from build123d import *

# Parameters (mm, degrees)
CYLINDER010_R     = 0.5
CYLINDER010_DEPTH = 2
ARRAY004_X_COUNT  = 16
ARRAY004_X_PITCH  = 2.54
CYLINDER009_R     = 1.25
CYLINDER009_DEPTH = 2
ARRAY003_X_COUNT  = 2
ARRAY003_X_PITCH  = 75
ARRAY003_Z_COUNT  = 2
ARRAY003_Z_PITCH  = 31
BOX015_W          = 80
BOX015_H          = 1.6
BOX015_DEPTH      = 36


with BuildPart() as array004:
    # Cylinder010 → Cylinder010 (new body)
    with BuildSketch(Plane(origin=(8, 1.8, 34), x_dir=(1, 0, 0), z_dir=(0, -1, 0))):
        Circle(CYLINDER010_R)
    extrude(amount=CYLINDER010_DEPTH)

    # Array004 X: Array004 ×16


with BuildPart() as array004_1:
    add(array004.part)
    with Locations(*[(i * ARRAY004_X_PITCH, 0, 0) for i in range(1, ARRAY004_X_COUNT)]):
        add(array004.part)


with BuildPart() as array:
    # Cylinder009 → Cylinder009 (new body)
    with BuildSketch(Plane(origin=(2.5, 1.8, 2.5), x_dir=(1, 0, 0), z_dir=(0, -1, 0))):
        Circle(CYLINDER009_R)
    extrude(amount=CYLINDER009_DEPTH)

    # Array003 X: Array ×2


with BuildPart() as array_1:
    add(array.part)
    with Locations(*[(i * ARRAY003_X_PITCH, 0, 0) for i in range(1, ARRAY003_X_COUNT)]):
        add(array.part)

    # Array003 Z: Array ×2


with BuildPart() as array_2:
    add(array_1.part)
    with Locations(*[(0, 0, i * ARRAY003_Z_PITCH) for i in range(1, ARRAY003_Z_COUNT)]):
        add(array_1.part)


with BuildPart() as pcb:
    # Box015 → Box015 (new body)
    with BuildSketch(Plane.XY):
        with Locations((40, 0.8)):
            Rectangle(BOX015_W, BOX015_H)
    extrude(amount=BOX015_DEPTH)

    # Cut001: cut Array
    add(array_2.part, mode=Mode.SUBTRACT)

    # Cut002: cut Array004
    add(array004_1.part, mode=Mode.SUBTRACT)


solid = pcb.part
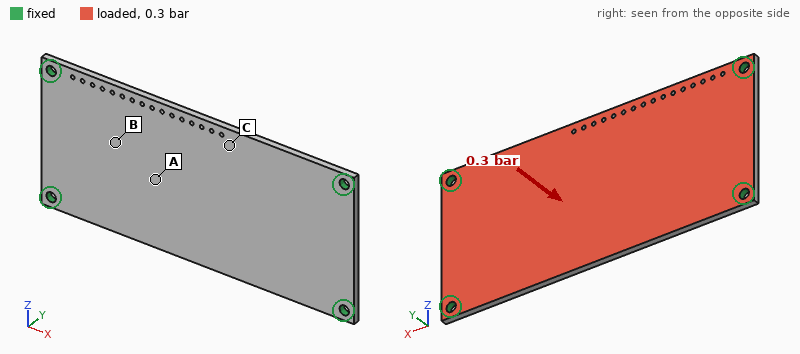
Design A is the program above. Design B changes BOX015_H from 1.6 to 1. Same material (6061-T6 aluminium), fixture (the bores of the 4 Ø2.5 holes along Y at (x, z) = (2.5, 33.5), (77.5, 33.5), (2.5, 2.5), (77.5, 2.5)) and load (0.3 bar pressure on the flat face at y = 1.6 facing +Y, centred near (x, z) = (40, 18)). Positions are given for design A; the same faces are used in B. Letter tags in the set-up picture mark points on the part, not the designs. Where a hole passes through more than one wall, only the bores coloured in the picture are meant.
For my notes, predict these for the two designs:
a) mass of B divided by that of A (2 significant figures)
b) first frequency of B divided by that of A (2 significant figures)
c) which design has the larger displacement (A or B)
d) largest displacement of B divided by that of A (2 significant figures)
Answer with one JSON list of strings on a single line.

["0.62", "0.64", "B", "4.0"]
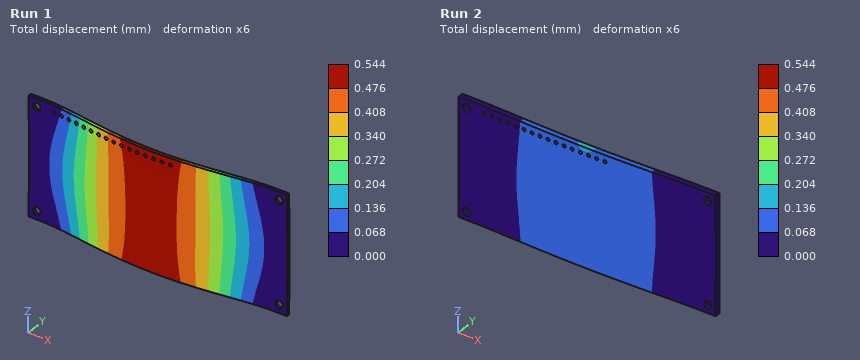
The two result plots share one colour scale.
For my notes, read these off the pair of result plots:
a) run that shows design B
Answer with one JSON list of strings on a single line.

["Run 1"]
